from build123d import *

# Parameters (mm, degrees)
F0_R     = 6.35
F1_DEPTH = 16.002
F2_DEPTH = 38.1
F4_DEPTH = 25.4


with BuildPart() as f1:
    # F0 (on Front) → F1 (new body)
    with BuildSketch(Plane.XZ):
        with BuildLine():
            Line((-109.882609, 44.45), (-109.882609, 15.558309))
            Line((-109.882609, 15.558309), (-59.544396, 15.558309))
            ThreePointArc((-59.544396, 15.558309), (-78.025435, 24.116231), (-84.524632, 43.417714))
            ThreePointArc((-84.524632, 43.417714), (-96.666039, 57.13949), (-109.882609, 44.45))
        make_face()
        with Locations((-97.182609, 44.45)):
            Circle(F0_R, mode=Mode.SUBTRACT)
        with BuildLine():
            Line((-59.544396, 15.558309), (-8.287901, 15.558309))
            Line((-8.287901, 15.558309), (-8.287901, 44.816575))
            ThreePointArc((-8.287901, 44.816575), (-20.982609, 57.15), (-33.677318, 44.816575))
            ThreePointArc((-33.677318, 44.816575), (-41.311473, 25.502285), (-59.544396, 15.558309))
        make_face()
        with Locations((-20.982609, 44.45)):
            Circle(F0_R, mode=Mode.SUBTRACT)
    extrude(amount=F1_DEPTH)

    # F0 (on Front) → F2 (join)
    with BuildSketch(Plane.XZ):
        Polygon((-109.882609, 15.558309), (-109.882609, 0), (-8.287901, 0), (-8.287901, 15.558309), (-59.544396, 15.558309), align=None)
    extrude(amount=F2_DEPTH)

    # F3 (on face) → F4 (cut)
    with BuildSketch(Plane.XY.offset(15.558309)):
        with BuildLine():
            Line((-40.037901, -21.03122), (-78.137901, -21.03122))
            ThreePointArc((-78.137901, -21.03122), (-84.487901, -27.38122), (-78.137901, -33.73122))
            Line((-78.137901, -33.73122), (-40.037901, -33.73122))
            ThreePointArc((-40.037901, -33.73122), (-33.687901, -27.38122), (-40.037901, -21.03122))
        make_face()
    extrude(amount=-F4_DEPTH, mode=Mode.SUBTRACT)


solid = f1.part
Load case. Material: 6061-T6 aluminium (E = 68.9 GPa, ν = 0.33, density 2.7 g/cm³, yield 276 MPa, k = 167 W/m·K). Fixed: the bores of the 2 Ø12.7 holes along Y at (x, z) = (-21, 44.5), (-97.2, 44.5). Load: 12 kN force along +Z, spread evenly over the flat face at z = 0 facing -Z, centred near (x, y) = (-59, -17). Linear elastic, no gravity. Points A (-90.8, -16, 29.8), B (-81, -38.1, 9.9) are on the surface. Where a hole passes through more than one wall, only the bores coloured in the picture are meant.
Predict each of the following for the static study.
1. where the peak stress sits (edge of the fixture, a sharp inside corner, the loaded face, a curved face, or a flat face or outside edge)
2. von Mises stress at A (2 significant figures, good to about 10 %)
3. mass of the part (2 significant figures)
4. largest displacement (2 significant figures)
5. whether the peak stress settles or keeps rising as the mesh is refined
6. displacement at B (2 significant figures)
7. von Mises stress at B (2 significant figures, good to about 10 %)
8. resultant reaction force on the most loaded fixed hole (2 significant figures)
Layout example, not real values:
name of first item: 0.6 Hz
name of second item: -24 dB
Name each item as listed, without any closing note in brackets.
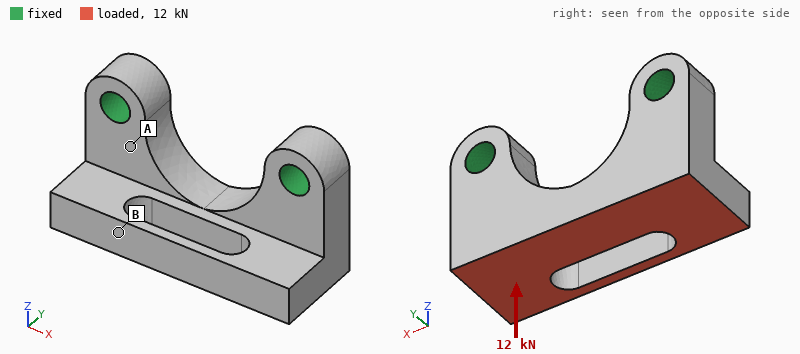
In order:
where the peak stress sits: edge of the fixture
von Mises stress at A: 63 MPa
mass of the part: 230 g
largest displacement: 0.13 mm
whether the peak stress settles or keeps rising as the mesh is refined: keeps rising
displacement at B: 0.11 mm
von Mises stress at B: 9.9 MPa
resultant reaction force on the most loaded fixed hole: 6.2 kN
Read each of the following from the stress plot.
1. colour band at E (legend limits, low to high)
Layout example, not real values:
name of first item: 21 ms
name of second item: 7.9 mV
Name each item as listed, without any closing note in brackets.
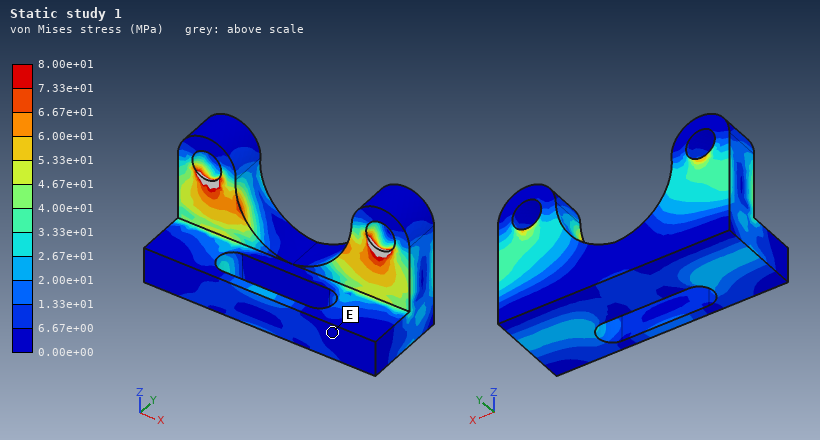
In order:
colour band at E: 0.00e+00 to 6.67e+00 MPa
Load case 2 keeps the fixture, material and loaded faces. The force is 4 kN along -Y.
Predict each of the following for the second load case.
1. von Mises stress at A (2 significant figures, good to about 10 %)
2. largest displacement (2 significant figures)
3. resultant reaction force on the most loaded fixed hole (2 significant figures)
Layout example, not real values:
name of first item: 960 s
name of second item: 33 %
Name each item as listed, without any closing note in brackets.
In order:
von Mises stress at A: 49 MPa
largest displacement: 0.13 mm
resultant reaction force on the most loaded fixed hole: 2.0 kN
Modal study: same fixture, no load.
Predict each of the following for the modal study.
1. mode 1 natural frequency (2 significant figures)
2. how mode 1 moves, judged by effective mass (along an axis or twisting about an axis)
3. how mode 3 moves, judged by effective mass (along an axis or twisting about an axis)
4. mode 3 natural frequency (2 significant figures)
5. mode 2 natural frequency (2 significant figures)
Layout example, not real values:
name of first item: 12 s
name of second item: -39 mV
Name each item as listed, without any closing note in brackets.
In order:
mode 1 natural frequency: 3400 Hz
how mode 1 moves, judged by effective mass: along Y
how mode 3 moves, judged by effective mass: along X
mode 3 natural frequency: 7600 Hz
mode 2 natural frequency: 5200 Hz
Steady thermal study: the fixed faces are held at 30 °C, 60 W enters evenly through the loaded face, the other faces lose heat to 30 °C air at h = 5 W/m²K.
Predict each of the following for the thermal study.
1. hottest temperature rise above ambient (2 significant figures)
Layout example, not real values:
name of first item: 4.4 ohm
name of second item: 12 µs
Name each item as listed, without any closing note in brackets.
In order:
hottest temperature rise above ambient: 17 K
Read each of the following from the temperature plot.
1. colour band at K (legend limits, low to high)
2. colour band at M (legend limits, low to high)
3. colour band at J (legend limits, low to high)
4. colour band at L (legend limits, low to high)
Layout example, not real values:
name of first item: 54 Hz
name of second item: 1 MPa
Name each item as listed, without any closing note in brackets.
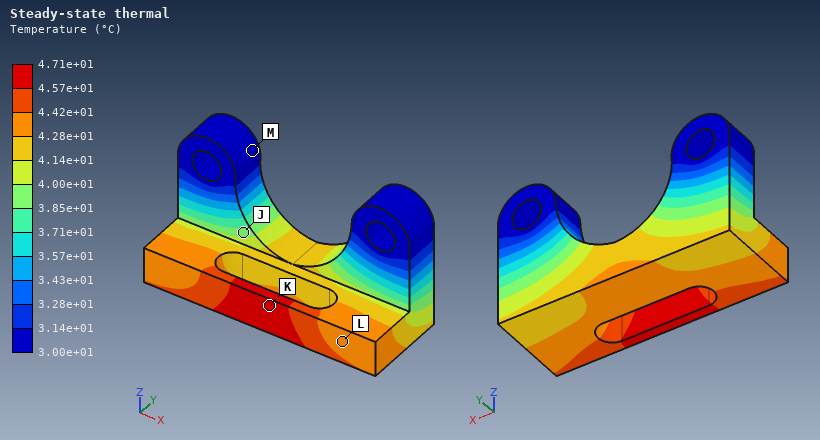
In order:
colour band at K: 4.57e+01 to 4.71e+01 °C
colour band at M: 3.00e+01 to 3.14e+01 °C
colour band at J: 3.85e+01 to 4.00e+01 °C
colour band at L: 4.28e+01 to 4.42e+01 °C
